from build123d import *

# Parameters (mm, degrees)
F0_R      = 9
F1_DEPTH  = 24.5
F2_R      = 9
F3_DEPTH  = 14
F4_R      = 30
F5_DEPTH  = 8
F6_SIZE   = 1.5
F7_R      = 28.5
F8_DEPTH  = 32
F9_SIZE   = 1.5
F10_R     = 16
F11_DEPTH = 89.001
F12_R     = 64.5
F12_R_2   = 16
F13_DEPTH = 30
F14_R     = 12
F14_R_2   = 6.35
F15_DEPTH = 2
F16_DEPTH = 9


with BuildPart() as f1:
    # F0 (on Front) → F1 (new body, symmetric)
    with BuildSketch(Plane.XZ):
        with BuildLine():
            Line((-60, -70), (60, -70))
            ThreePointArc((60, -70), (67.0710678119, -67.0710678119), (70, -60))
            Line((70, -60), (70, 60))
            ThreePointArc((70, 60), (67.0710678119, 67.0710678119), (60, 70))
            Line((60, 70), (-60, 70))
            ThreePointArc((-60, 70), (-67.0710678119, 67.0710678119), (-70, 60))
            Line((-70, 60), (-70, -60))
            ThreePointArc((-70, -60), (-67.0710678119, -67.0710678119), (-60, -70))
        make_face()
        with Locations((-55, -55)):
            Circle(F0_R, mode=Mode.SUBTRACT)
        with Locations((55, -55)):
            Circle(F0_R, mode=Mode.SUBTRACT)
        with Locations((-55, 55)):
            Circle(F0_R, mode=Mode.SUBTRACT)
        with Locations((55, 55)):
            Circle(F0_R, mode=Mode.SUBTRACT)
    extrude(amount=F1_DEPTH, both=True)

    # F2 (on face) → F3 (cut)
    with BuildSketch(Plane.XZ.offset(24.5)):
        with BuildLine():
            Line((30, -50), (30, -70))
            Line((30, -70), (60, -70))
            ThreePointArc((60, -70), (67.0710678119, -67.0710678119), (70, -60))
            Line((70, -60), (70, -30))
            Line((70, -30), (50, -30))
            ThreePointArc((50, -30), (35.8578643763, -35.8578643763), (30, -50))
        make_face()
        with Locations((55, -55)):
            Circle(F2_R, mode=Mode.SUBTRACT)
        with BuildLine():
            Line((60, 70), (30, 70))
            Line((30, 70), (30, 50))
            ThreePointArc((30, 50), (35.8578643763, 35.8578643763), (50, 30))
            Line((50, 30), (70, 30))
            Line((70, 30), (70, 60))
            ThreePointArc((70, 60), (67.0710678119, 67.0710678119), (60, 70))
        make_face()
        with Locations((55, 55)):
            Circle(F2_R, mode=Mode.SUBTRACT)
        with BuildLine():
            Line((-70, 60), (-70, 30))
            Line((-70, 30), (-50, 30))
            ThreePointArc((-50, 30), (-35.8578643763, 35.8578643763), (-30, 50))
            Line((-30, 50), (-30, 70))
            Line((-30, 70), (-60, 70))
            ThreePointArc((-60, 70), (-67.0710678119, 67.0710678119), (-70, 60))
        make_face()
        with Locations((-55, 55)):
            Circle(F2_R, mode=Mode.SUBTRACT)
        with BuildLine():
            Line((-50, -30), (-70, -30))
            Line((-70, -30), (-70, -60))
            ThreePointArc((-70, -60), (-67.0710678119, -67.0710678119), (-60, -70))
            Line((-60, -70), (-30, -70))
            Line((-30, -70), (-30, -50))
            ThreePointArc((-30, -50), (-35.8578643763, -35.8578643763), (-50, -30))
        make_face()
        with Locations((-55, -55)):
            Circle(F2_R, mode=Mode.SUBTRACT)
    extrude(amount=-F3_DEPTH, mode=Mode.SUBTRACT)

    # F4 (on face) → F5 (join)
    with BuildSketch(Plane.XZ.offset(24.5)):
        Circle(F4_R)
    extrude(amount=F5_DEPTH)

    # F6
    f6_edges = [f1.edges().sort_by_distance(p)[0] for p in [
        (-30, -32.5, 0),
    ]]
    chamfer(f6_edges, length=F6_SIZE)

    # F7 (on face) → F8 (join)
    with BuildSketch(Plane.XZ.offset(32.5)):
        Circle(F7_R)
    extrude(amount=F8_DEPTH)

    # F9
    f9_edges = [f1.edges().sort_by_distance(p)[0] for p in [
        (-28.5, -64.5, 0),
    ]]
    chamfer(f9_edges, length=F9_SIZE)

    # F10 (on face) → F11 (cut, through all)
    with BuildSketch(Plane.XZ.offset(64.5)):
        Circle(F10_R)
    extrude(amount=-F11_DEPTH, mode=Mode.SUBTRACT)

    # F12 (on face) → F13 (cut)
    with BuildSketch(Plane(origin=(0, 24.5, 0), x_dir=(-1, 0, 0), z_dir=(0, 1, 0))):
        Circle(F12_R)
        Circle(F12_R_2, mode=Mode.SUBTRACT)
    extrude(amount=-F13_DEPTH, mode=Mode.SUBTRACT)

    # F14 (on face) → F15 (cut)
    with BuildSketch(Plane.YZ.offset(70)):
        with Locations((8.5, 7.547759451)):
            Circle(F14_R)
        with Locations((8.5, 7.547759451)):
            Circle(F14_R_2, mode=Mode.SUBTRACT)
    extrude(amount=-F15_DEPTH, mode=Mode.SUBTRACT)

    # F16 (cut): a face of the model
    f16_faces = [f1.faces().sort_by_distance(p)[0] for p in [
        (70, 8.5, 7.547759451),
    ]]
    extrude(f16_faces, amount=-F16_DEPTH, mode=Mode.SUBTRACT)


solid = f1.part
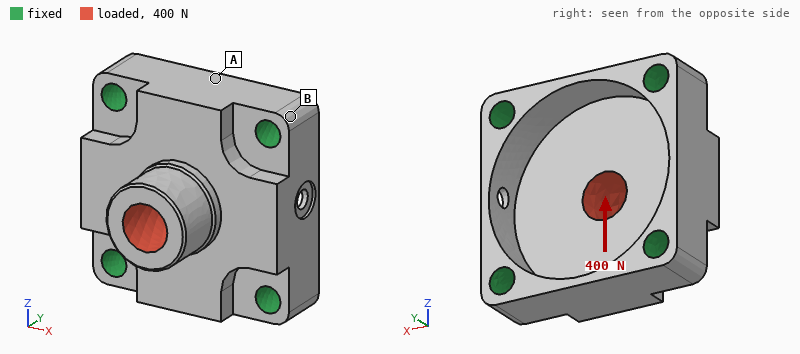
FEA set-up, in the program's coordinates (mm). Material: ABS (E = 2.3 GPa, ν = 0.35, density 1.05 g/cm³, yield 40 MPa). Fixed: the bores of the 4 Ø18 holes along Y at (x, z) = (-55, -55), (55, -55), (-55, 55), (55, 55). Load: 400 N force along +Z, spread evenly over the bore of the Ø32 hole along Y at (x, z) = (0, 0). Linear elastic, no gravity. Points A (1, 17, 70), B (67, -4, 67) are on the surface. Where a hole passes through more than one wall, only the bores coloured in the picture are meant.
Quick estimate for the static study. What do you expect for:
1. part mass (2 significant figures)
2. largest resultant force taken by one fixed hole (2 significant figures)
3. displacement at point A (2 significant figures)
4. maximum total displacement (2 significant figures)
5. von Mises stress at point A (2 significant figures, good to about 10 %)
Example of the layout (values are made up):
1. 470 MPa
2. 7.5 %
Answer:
1. 520 g
2. 130 N
3. 4.2 µm
4. 27 µm
5. 0.12 MPa
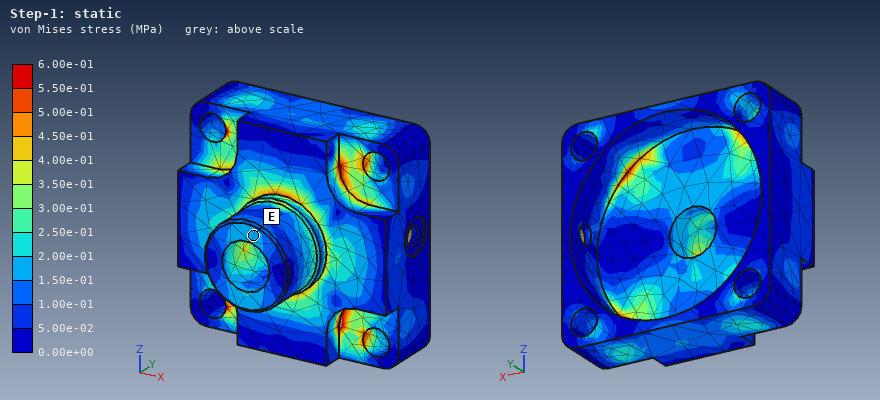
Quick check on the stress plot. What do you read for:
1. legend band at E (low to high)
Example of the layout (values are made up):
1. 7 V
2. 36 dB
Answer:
1. 1.50e-01 to 2.00e-01 MPa
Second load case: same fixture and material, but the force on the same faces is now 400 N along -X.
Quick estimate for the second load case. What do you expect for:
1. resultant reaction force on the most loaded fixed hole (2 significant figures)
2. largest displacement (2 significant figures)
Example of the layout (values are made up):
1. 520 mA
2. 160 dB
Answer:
1. 130 N
2. 27 µm
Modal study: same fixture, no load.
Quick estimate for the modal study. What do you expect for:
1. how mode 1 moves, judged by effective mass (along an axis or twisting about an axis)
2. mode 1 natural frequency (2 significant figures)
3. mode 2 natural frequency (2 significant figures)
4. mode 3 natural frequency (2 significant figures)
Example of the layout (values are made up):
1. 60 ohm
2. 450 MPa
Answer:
1. along Y
2. 1400 Hz
3. 1900 Hz
4. 1900 Hz
